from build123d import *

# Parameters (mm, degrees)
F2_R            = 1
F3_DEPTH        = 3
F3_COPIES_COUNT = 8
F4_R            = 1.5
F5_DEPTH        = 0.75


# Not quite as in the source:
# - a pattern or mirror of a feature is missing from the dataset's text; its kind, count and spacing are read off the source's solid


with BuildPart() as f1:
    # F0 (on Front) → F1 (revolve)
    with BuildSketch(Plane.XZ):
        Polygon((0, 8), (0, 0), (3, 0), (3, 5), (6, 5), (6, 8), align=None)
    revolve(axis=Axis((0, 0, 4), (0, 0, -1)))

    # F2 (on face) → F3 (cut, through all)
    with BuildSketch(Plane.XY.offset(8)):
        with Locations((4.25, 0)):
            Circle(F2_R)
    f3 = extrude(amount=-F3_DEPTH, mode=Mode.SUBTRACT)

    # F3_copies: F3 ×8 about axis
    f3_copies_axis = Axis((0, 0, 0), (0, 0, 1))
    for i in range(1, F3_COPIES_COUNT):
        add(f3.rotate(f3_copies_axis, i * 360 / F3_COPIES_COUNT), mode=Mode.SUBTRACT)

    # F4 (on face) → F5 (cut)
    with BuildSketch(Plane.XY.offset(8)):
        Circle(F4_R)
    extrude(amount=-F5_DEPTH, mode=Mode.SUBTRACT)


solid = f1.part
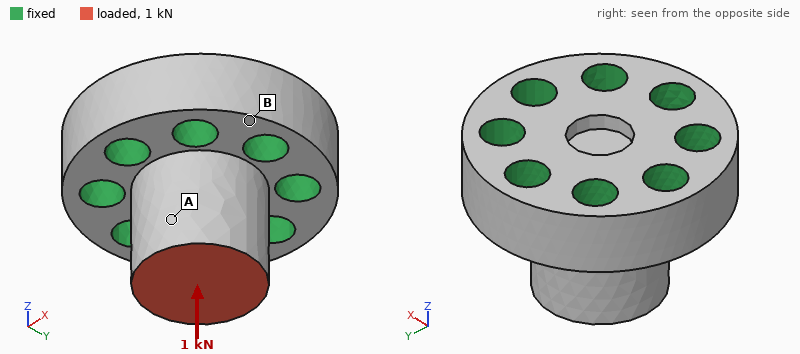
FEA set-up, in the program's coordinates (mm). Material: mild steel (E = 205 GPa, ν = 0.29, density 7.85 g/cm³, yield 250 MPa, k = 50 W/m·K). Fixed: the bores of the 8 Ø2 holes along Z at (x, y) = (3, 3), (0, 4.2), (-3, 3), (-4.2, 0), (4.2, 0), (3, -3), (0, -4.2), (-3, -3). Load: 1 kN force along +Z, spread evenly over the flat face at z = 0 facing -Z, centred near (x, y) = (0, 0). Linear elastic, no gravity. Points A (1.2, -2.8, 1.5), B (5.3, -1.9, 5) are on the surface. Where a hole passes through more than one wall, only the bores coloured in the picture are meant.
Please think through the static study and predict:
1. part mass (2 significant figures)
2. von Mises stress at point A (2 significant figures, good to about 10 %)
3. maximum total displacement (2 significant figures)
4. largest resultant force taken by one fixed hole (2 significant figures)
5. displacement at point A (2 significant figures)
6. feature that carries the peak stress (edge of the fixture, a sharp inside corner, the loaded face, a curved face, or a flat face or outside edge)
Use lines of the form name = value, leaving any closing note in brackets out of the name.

part mass = 3.1 g
von Mises stress at point A = 35 MPa
maximum total displacement = 1.2 µm
largest resultant force taken by one fixed hole = 140 N
displacement at point A = 0.95 µm
feature that carries the peak stress = edge of the fixture
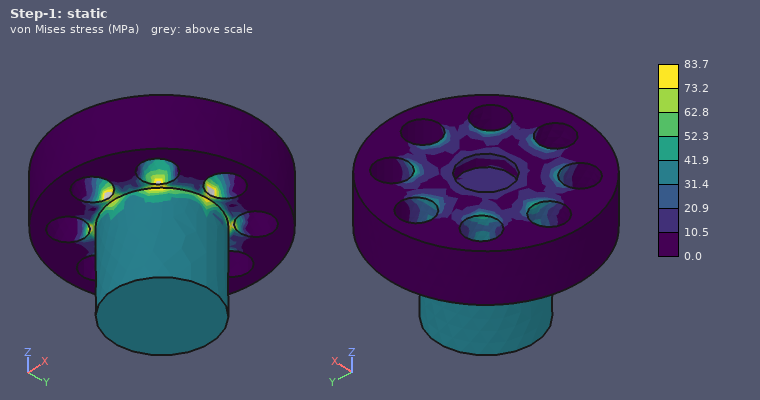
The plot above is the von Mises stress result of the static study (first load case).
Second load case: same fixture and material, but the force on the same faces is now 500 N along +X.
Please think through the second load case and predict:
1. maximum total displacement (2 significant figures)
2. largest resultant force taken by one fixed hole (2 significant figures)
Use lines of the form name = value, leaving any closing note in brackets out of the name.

maximum total displacement = 4.6 µm
largest resultant force taken by one fixed hole = 250 N
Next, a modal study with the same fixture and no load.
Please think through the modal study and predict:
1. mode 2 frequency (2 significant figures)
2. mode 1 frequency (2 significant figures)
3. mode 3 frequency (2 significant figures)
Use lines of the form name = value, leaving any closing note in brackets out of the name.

mode 2 frequency = 89 kHz
mode 1 frequency = 89 kHz
mode 3 frequency = 140 kHz
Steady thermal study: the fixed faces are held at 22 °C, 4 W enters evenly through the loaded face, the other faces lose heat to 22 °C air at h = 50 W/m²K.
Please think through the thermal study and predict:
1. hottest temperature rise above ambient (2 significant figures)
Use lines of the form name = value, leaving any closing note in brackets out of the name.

hottest temperature rise above ambient = 17 K
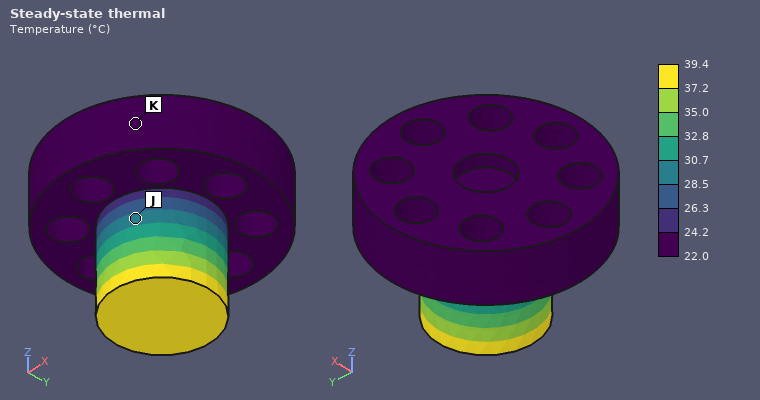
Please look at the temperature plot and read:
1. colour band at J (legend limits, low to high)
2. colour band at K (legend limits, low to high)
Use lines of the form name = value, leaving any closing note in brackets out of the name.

colour band at J = 28.5 to 30.7 °C
colour band at K = 22.0 to 24.2 °C
